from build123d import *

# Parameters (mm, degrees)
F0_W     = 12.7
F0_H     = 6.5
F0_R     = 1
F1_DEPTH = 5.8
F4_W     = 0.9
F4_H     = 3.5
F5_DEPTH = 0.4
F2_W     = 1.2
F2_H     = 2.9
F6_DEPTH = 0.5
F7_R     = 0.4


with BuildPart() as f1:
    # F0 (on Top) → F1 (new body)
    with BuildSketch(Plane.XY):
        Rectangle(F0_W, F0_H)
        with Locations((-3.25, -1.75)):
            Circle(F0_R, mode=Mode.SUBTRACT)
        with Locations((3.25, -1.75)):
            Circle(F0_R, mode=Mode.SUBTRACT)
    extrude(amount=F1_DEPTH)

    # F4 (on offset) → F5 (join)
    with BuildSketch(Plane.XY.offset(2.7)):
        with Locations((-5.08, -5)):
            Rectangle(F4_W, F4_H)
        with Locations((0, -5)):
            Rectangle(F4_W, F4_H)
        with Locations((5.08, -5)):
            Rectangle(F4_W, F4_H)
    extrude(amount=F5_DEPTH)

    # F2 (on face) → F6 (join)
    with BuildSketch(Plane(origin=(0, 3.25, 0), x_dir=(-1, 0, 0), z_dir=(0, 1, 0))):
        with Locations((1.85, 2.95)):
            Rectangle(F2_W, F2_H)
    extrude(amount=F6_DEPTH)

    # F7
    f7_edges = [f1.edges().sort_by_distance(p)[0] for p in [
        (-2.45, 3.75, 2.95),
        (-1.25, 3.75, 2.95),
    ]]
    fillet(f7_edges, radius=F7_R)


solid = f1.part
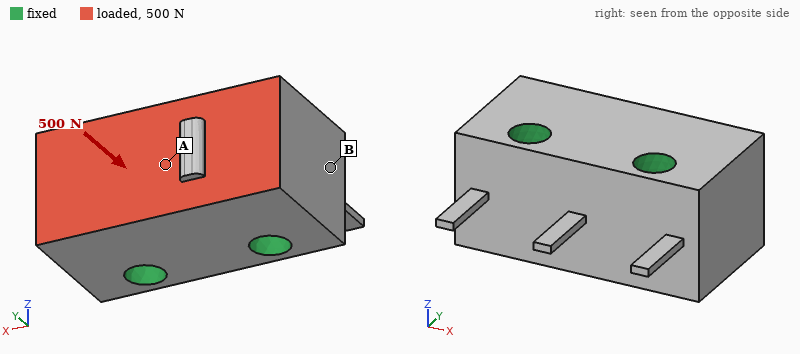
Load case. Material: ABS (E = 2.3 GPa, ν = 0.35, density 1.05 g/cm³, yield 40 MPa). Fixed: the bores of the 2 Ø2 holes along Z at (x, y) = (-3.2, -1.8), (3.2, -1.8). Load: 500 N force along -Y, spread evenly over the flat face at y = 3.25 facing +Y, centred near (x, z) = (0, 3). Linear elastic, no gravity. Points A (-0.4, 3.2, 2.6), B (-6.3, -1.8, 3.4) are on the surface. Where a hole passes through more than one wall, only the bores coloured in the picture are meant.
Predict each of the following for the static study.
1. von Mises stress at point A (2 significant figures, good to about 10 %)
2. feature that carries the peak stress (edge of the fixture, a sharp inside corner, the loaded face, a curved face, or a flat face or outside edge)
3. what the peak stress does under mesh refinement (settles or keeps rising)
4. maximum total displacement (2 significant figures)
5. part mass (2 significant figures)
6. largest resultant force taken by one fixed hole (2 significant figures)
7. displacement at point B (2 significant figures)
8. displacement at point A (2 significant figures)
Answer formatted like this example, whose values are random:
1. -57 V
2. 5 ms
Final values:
1. 7.1 MPa
2. edge of the fixture
3. keeps rising
4. 24 µm
5. 0.47 g
6. 260 N
7. 10 µm
8. 14 µm
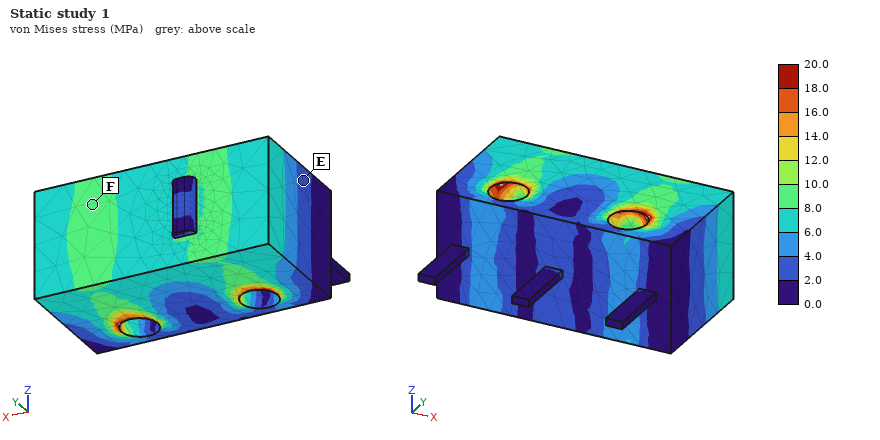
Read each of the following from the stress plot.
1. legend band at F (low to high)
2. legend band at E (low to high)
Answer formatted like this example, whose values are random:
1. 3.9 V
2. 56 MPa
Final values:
1. 8.0 to 10.0 MPa
2. 2.0 to 4.0 MPa
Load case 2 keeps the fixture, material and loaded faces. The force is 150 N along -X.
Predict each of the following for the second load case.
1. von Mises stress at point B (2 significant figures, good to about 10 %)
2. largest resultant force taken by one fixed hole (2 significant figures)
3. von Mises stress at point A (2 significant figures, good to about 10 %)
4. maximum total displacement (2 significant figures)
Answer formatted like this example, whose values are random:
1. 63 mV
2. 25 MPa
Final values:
1. 1.6 MPa
2. 110 N
3. 3.7 MPa
4. 28 µm
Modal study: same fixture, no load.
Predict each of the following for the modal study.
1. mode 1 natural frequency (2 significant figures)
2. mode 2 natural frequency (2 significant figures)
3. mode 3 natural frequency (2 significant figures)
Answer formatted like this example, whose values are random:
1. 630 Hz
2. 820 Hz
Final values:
1. 7500 Hz
2. 7500 Hz
3. 7500 Hz
